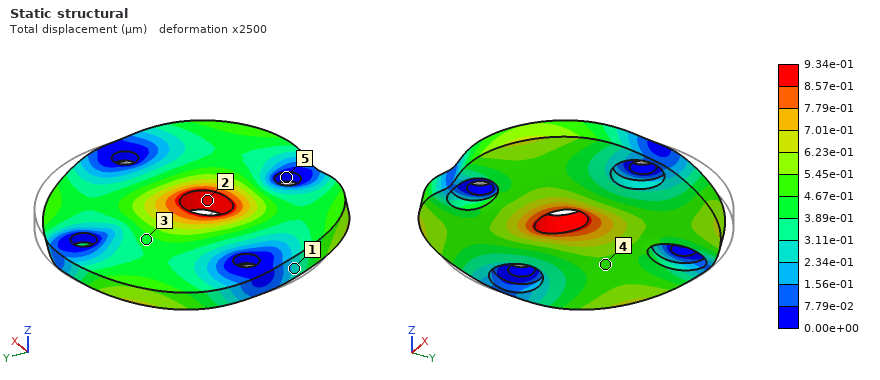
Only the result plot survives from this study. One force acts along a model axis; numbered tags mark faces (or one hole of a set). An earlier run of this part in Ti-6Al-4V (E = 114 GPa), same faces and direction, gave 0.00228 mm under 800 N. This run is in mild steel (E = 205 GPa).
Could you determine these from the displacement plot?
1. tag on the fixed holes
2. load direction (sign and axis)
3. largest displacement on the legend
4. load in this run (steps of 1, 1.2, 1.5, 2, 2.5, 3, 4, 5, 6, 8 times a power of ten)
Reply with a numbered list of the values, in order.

1. 5
2. -Y
3. 9.34e-01 µm
4. 600 N
